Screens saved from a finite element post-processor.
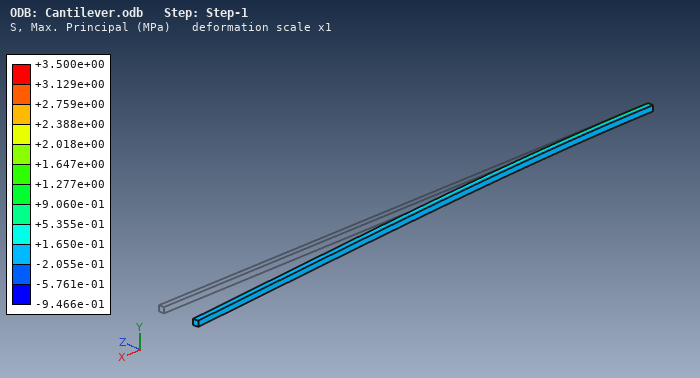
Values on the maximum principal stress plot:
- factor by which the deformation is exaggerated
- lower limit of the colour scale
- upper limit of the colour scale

1
-9.466e-01 MPa
+3.500e+00 MPa
